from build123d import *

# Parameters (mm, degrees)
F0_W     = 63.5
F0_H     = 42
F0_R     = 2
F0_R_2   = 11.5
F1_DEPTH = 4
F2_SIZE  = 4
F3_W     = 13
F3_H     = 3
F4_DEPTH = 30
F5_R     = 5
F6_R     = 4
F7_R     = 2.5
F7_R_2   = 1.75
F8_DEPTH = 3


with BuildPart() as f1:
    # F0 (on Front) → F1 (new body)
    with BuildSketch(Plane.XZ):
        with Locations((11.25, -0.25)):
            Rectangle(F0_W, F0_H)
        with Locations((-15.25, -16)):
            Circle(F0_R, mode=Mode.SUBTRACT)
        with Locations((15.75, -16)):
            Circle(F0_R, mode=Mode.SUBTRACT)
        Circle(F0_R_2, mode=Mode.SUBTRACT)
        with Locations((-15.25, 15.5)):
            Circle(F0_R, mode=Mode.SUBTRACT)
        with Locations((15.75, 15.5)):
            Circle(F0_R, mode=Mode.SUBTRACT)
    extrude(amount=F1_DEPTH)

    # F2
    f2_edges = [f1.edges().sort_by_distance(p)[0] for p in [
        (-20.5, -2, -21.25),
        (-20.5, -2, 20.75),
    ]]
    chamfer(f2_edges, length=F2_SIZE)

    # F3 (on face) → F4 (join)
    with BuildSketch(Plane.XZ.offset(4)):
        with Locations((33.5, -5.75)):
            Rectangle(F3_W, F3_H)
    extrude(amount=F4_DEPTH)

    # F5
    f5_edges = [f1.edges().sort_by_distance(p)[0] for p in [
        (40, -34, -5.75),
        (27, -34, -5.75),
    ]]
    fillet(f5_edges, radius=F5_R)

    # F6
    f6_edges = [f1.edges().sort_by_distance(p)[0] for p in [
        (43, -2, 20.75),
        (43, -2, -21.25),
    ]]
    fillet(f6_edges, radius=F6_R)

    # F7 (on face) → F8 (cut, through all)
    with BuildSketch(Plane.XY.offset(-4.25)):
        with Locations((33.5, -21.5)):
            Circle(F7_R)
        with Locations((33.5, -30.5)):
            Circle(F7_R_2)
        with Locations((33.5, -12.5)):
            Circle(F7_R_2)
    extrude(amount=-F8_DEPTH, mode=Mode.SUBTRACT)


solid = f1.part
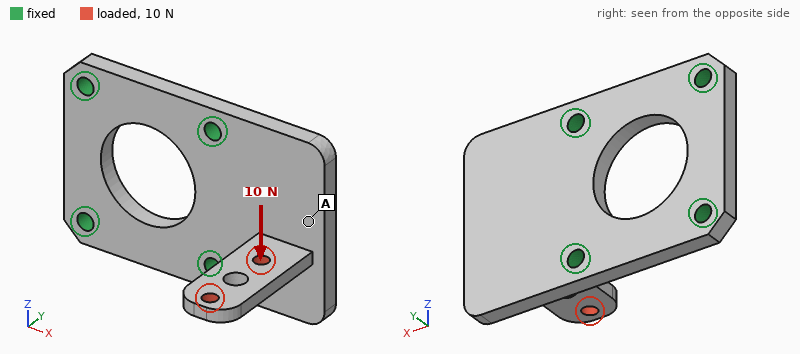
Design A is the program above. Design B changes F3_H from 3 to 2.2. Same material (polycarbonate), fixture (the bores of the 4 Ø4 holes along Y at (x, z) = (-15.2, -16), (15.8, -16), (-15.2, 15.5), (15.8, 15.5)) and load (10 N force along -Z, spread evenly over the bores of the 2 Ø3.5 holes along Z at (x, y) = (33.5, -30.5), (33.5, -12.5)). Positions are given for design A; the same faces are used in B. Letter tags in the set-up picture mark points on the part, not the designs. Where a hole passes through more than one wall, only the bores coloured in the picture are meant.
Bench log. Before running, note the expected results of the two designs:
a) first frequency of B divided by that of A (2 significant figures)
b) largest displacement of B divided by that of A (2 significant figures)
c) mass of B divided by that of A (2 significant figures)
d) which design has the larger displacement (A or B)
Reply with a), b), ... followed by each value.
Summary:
a) 0.78
b) 2.3
c) 0.97
d) B
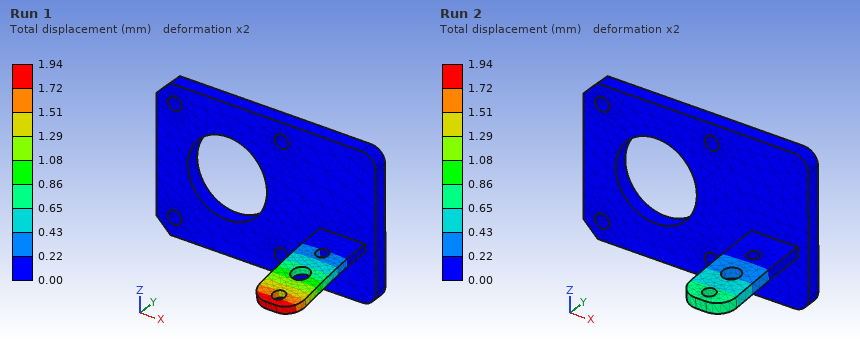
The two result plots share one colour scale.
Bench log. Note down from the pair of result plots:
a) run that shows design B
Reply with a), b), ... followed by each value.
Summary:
a) Run 1
